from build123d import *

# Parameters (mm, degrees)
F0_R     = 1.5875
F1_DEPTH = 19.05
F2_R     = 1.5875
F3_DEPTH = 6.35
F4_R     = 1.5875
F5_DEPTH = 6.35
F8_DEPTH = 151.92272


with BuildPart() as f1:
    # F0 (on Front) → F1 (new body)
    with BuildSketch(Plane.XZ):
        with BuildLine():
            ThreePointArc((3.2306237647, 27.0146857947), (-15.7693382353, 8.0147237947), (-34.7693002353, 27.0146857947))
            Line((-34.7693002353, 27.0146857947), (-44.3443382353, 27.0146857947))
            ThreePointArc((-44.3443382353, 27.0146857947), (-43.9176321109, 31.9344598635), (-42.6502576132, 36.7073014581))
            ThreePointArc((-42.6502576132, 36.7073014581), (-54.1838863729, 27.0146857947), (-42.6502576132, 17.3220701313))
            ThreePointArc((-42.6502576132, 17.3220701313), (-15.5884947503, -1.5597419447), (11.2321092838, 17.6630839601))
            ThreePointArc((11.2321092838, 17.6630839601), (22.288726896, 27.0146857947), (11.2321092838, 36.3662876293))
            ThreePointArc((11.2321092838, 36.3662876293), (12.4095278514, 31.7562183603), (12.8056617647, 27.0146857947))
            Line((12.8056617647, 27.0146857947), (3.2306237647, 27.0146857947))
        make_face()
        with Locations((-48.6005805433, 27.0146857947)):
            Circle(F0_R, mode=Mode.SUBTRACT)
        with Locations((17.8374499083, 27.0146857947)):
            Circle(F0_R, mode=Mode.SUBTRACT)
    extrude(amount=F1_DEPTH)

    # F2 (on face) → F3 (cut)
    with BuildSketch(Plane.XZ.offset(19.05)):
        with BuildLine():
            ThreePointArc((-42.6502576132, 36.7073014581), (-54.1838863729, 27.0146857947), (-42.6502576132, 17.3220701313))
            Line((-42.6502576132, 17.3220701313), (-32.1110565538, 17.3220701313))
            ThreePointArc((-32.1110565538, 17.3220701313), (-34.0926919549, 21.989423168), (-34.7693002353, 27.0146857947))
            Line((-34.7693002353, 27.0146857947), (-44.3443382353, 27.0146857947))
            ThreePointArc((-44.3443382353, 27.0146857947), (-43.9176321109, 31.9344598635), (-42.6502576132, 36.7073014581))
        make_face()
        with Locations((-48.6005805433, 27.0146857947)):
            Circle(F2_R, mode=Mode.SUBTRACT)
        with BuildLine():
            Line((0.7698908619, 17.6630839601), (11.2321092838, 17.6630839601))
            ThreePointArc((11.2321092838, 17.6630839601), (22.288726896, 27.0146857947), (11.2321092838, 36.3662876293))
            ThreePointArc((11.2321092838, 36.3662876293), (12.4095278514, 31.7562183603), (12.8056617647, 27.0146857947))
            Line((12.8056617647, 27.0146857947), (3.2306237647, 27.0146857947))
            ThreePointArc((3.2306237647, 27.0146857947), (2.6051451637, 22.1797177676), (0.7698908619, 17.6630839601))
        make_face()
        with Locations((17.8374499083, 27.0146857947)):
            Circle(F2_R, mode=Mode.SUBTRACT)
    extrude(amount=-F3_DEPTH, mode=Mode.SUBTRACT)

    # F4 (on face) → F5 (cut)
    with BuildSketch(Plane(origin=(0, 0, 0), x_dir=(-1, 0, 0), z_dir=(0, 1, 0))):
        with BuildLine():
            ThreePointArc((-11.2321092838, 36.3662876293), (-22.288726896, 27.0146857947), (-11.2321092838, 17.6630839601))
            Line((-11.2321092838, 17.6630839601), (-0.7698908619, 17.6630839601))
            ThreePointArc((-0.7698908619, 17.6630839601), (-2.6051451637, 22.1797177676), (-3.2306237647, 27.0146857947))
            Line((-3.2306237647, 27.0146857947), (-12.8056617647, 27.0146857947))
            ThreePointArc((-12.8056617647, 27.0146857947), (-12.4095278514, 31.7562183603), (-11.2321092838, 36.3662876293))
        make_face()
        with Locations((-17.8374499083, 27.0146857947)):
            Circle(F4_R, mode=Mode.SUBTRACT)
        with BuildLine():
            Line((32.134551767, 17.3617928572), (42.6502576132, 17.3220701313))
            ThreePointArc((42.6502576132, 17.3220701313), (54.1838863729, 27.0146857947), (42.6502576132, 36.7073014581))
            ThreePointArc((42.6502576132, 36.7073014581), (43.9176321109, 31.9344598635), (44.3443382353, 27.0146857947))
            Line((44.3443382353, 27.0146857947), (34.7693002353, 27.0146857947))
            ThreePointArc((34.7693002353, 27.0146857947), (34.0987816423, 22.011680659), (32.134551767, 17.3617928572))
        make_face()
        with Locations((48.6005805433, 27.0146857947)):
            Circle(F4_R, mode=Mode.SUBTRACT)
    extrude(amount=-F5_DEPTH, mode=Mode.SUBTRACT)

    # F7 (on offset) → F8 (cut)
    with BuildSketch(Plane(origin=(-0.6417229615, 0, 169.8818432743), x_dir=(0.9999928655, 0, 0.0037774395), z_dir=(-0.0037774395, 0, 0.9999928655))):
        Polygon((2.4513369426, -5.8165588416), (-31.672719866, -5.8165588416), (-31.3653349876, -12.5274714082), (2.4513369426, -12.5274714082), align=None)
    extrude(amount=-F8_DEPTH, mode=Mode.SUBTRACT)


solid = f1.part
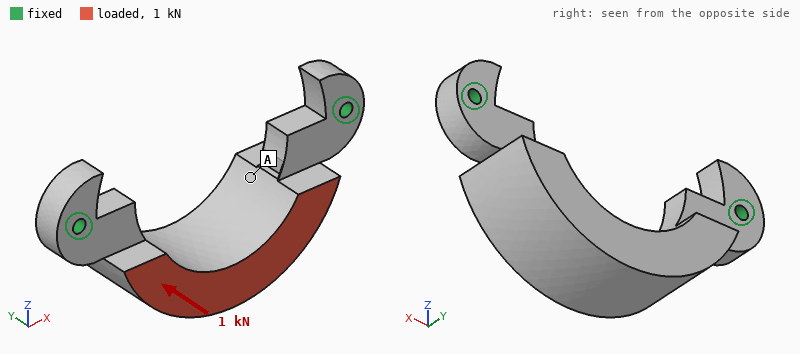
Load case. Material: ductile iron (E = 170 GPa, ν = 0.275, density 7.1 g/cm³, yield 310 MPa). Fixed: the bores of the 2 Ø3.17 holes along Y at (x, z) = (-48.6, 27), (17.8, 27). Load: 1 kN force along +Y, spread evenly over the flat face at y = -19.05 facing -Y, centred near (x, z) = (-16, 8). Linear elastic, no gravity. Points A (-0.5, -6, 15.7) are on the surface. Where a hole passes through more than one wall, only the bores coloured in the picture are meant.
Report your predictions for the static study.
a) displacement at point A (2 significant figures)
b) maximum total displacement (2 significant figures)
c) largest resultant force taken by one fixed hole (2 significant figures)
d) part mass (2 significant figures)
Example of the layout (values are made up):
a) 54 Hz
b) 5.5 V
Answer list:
a) 31 µm
b) 94 µm
c) 500 N
d) 93 g
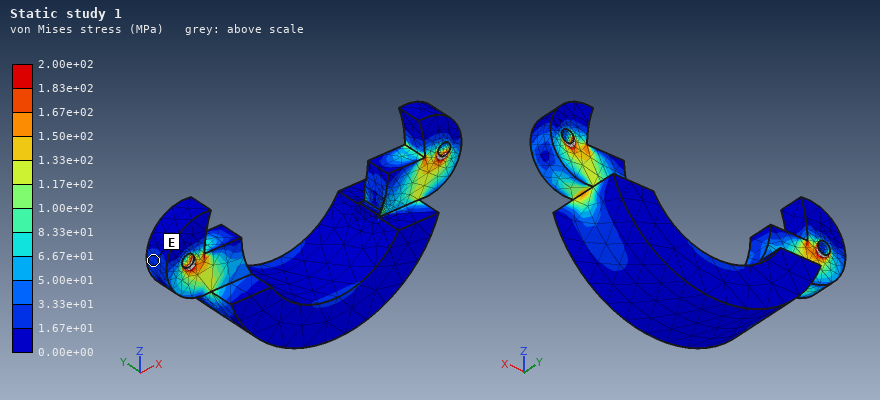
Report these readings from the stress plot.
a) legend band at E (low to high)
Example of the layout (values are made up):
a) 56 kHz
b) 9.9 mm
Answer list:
a) 1.67e+01 to 3.33e+01 MPa
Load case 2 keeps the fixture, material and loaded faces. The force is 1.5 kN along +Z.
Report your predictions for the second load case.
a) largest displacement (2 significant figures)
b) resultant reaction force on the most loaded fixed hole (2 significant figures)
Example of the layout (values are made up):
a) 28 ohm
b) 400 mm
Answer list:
a) 92 µm
b) 970 N
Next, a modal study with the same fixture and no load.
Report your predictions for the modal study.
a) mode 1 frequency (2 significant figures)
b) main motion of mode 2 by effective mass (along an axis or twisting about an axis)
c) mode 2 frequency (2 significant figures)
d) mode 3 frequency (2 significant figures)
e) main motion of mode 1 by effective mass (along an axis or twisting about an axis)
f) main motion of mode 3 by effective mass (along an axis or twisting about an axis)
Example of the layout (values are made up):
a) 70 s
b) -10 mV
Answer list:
a) 2300 Hz
b) along X
c) 9600 Hz
d) 11 kHz
e) along Y
f) twisting about Z
